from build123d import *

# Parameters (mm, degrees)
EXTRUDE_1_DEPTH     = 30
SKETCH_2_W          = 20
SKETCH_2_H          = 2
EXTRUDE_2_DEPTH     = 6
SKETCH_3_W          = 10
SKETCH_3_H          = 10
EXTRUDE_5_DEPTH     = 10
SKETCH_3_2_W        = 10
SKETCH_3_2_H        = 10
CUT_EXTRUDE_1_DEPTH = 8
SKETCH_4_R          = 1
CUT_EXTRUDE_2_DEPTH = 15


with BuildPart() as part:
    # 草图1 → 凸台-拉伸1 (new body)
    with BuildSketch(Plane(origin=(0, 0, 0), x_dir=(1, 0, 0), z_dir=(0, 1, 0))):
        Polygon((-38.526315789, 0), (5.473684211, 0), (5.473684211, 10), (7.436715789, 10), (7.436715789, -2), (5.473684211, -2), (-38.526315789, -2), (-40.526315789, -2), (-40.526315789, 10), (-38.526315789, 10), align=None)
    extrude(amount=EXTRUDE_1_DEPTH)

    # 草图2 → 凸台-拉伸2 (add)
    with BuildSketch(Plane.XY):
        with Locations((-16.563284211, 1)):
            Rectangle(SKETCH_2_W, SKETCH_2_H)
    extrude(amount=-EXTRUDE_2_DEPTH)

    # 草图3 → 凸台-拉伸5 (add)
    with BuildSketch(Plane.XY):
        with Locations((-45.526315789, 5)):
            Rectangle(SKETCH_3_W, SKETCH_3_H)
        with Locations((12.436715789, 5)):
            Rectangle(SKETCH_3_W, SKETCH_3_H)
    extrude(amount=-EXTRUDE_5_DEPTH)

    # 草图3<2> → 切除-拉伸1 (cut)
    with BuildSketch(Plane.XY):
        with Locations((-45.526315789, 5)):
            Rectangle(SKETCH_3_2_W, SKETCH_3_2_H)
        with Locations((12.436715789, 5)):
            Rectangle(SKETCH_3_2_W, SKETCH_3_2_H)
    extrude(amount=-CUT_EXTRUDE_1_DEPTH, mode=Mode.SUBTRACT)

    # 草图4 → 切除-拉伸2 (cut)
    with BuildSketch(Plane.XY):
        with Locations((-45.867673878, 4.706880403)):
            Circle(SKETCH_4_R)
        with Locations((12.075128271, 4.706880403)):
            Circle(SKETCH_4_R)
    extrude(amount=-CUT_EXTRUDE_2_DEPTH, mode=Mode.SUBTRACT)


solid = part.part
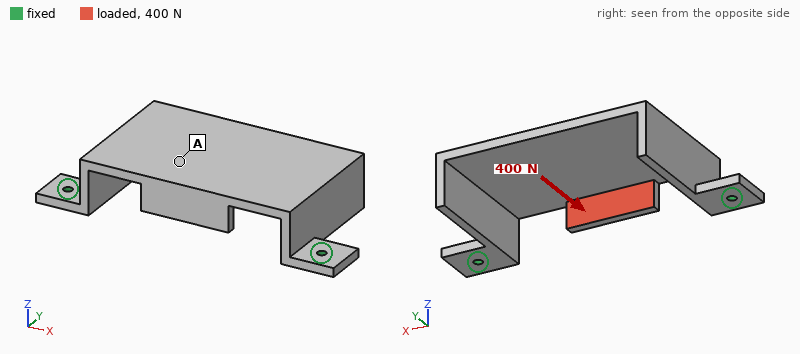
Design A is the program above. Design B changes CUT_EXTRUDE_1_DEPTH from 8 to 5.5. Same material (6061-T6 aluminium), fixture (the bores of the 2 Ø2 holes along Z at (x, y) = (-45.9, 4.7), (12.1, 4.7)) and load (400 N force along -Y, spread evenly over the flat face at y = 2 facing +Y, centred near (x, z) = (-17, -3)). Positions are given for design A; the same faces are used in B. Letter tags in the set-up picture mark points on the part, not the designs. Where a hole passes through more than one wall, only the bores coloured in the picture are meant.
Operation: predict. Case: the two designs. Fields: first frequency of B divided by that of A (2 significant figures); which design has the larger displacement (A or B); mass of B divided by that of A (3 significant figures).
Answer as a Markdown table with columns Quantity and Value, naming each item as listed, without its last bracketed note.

| Quantity | Value |
|---|---|
| first frequency of B divided by that of A | 2.0 |
| which design has the larger displacement | A |
| mass of B divided by that of A | 1.10 |
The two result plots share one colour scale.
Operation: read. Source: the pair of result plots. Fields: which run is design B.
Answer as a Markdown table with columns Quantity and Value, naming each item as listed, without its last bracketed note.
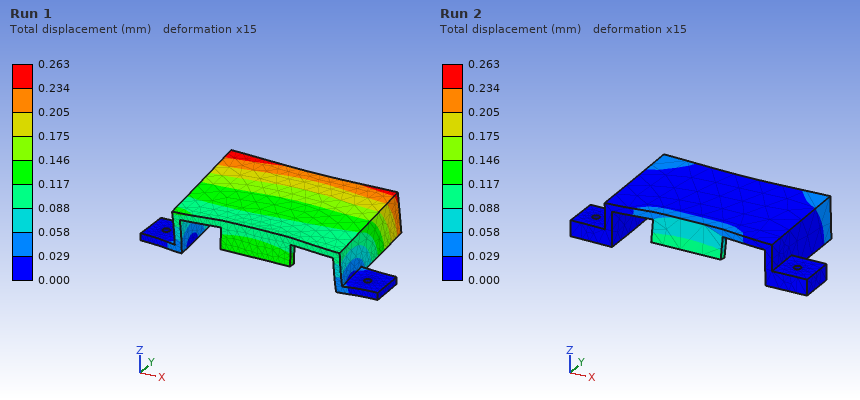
| Quantity | Value |
|---|---|
| which run is design B | Run 2 |
